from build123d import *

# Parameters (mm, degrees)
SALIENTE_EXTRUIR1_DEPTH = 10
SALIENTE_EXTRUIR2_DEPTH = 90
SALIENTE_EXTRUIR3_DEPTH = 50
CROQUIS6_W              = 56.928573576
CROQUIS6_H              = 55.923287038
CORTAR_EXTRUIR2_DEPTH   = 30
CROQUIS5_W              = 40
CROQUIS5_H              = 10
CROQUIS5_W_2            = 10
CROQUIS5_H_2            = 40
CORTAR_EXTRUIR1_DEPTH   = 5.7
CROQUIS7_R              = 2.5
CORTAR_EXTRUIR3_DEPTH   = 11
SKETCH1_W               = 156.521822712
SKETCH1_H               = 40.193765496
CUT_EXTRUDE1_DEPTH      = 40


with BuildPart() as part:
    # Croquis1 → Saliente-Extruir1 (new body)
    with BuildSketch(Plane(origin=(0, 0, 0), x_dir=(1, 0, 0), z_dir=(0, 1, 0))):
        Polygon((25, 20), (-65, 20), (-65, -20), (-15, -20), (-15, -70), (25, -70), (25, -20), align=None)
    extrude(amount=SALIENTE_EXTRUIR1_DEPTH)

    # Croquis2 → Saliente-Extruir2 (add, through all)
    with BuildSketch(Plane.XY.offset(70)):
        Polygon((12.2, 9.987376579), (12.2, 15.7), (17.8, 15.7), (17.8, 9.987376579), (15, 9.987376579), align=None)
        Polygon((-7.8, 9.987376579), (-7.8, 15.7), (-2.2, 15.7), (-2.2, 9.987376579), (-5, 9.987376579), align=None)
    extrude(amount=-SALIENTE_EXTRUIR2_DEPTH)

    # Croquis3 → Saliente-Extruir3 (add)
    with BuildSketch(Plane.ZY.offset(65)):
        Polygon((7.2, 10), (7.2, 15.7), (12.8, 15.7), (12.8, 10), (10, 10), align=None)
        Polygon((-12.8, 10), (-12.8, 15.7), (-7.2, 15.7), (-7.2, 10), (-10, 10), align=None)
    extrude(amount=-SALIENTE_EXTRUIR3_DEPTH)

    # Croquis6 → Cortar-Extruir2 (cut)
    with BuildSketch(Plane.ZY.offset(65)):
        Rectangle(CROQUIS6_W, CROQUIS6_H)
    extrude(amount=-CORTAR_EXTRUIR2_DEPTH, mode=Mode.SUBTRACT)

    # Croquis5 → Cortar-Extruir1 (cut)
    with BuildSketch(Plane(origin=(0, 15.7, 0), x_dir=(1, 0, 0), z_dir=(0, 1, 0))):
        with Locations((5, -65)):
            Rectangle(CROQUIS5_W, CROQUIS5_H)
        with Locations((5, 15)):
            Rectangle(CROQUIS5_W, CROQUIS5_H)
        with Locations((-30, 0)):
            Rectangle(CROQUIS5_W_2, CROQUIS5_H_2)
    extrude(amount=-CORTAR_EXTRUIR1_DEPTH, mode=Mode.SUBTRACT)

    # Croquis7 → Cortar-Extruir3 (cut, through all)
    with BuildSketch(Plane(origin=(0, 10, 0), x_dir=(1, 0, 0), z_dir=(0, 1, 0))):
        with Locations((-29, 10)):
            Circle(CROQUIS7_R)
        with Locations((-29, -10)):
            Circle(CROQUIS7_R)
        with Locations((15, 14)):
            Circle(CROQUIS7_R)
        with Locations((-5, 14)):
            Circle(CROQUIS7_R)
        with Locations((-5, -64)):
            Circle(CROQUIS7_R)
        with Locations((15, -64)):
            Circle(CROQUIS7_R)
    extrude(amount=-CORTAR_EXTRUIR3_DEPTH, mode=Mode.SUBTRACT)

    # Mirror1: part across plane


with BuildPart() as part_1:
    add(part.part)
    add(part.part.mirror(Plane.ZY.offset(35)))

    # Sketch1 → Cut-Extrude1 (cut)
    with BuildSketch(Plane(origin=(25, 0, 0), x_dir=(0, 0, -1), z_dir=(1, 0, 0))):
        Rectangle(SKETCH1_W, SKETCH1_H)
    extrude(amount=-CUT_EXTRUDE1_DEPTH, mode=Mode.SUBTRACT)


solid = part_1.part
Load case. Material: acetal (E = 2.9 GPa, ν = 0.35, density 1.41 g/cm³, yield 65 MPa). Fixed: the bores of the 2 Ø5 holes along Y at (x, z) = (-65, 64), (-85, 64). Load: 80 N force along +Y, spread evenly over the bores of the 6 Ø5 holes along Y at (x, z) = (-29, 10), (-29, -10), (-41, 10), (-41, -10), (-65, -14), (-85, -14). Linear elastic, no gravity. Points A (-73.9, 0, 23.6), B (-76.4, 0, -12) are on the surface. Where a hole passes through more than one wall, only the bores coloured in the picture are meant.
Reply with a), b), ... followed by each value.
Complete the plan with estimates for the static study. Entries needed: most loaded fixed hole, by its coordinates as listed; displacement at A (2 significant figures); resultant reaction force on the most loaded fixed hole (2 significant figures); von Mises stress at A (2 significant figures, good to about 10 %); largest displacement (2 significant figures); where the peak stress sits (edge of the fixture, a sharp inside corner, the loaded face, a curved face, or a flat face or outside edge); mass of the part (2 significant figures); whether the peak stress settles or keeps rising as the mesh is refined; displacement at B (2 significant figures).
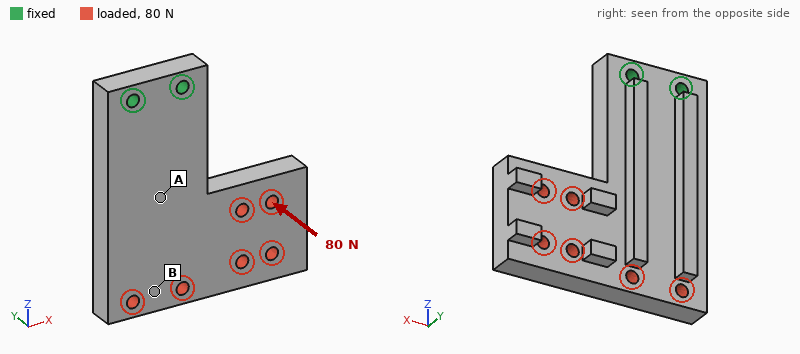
a) (-65, 64)
b) 0.30 mm
c) 110 N
d) 3.0 MPa
e) 1.4 mm
f) edge of the fixture
g) 79 g
h) keeps rising
i) 0.69 mm
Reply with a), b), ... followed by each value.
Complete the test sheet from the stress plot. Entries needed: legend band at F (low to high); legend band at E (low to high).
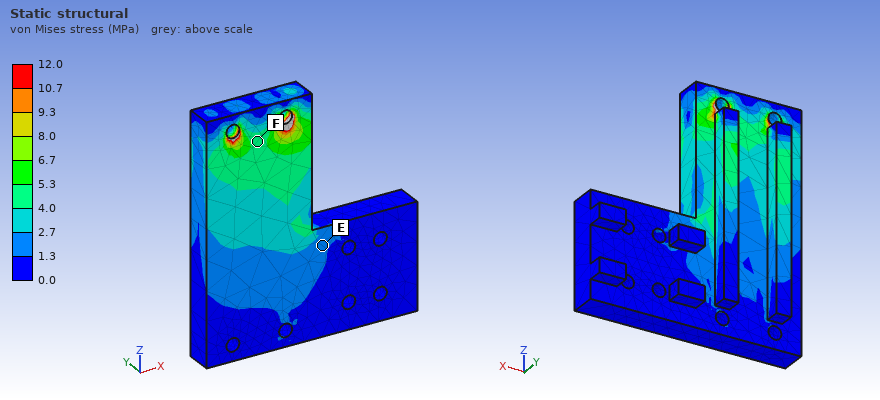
a) 4.0 to 5.3 MPa
b) 1.3 to 2.7 MPa
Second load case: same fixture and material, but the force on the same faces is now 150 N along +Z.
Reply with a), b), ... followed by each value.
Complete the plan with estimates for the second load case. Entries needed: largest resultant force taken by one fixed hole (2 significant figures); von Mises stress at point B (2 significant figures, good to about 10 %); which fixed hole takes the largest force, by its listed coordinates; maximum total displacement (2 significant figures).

a) 250 N
b) 0.35 MPa
c) (-65, 64)
d) 0.16 mm
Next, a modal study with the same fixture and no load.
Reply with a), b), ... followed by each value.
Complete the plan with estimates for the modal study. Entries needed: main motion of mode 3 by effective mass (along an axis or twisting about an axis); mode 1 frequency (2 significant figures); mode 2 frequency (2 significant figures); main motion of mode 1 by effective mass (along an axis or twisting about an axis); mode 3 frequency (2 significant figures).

a) along X
b) 240 Hz
c) 530 Hz
d) along Y
e) 650 Hz
